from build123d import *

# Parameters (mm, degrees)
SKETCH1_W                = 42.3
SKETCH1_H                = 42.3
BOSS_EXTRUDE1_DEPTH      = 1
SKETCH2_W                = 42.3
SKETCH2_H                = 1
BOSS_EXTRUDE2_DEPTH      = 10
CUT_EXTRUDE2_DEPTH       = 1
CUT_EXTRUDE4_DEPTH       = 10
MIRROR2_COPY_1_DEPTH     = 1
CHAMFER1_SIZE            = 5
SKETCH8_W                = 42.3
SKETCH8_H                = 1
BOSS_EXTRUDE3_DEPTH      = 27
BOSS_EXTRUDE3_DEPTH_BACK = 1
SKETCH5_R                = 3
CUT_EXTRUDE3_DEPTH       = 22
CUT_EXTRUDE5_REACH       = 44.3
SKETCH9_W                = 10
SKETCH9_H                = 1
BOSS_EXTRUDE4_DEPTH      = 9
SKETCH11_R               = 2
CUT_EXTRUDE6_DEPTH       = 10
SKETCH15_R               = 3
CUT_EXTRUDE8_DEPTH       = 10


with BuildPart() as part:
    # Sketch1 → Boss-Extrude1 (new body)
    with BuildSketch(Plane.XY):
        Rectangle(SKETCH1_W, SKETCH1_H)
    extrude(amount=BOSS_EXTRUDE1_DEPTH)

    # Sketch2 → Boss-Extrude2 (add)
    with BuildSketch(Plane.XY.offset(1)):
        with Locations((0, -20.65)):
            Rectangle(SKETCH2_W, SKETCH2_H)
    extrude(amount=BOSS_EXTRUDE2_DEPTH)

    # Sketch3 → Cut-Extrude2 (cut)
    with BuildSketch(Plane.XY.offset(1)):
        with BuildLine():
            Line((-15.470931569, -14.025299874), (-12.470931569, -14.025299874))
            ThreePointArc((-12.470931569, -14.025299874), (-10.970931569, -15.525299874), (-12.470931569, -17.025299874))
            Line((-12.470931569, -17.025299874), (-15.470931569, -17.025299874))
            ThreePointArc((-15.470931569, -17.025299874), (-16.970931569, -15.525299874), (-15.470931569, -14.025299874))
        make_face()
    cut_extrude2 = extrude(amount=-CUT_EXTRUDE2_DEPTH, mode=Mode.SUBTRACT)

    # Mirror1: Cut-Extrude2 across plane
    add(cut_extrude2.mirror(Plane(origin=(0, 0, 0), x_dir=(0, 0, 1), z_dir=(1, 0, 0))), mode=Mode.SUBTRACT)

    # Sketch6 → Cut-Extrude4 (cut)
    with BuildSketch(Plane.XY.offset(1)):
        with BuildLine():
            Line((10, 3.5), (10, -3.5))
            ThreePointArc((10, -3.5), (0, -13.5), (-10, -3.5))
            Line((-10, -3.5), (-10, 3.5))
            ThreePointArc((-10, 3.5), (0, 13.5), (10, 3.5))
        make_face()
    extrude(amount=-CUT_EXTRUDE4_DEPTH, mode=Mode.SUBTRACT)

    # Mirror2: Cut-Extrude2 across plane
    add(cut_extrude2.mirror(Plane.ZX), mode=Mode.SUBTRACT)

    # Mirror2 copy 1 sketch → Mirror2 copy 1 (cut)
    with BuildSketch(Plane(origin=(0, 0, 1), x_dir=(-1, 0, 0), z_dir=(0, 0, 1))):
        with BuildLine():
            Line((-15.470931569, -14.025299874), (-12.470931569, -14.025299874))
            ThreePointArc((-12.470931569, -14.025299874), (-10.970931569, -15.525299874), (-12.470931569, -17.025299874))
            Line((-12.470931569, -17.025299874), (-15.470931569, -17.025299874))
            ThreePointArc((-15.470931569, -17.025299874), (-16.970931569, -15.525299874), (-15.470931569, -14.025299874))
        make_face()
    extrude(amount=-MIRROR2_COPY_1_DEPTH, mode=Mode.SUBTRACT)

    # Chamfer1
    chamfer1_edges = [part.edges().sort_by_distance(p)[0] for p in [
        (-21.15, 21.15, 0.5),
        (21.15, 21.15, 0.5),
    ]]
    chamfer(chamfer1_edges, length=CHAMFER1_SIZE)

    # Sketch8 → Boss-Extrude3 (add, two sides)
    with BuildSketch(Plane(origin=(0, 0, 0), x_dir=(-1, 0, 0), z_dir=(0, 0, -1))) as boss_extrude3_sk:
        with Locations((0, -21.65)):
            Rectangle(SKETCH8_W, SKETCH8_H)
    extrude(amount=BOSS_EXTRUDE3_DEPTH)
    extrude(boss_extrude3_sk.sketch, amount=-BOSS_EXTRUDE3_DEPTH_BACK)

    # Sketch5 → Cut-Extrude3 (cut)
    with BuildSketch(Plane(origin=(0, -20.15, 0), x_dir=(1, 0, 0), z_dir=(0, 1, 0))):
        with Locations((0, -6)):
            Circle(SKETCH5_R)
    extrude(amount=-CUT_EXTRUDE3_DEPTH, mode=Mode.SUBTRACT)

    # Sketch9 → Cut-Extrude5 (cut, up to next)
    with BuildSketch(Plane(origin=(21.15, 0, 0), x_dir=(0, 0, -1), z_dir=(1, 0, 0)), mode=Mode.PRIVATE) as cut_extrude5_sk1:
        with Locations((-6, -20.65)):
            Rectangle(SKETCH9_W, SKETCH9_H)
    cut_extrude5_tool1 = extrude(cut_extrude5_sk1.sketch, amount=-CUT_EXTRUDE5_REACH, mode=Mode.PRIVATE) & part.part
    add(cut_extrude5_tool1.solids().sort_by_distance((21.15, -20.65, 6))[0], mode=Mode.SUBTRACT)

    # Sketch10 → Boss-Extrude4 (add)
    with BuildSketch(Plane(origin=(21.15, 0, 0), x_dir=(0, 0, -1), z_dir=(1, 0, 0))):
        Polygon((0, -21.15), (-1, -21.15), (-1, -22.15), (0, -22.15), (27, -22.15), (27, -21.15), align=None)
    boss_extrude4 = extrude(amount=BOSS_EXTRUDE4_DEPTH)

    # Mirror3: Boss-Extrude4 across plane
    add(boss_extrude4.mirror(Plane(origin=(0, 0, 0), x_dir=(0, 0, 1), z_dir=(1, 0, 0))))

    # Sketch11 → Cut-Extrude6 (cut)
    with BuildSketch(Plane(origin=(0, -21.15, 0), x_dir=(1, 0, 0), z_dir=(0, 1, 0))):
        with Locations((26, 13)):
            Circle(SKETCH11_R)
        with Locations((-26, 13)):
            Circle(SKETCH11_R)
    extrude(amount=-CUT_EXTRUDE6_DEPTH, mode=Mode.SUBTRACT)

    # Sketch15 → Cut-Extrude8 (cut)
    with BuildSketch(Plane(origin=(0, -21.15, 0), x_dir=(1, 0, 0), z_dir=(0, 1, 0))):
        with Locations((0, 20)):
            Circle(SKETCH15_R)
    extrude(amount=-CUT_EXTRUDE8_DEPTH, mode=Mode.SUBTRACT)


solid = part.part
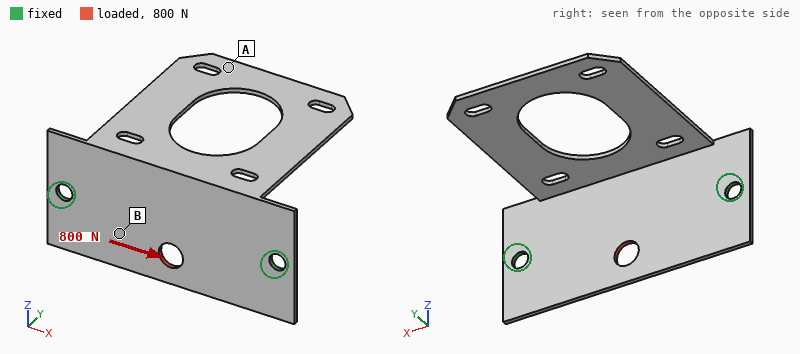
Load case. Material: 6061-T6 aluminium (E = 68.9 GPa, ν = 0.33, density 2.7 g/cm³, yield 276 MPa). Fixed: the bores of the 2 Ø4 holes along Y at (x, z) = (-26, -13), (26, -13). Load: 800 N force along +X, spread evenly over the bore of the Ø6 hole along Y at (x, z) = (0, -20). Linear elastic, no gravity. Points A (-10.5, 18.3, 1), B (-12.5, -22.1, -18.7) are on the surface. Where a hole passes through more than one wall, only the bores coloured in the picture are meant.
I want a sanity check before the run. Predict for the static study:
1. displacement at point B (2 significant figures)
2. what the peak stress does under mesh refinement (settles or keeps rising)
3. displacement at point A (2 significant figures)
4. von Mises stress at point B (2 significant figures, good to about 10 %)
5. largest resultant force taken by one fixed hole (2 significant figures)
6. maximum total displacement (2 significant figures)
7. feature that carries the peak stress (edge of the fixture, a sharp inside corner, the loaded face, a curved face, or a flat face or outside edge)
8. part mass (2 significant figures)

6.9 µm
keeps rising
4.1 µm
29 MPa
410 N
14 µm
edge of the fixture
7.8 g
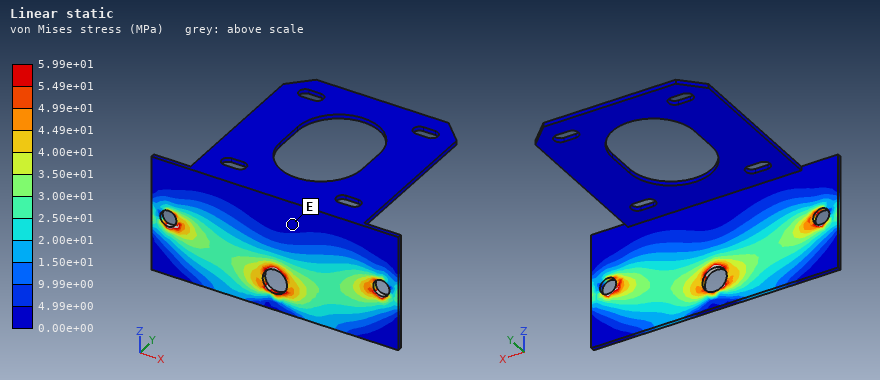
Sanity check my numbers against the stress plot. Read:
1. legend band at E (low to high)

0.00e+00 to 4.99e+00 MPa
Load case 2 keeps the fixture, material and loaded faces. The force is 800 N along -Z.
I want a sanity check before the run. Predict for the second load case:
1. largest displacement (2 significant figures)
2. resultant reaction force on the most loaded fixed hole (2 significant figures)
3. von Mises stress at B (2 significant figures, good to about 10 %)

42 µm
400 N
29 MPa
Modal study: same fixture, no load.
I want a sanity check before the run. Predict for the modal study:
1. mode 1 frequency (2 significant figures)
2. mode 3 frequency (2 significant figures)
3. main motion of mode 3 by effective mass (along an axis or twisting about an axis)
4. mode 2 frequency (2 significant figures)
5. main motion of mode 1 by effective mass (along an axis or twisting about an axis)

320 Hz
1300 Hz
along X
880 Hz
along Z
